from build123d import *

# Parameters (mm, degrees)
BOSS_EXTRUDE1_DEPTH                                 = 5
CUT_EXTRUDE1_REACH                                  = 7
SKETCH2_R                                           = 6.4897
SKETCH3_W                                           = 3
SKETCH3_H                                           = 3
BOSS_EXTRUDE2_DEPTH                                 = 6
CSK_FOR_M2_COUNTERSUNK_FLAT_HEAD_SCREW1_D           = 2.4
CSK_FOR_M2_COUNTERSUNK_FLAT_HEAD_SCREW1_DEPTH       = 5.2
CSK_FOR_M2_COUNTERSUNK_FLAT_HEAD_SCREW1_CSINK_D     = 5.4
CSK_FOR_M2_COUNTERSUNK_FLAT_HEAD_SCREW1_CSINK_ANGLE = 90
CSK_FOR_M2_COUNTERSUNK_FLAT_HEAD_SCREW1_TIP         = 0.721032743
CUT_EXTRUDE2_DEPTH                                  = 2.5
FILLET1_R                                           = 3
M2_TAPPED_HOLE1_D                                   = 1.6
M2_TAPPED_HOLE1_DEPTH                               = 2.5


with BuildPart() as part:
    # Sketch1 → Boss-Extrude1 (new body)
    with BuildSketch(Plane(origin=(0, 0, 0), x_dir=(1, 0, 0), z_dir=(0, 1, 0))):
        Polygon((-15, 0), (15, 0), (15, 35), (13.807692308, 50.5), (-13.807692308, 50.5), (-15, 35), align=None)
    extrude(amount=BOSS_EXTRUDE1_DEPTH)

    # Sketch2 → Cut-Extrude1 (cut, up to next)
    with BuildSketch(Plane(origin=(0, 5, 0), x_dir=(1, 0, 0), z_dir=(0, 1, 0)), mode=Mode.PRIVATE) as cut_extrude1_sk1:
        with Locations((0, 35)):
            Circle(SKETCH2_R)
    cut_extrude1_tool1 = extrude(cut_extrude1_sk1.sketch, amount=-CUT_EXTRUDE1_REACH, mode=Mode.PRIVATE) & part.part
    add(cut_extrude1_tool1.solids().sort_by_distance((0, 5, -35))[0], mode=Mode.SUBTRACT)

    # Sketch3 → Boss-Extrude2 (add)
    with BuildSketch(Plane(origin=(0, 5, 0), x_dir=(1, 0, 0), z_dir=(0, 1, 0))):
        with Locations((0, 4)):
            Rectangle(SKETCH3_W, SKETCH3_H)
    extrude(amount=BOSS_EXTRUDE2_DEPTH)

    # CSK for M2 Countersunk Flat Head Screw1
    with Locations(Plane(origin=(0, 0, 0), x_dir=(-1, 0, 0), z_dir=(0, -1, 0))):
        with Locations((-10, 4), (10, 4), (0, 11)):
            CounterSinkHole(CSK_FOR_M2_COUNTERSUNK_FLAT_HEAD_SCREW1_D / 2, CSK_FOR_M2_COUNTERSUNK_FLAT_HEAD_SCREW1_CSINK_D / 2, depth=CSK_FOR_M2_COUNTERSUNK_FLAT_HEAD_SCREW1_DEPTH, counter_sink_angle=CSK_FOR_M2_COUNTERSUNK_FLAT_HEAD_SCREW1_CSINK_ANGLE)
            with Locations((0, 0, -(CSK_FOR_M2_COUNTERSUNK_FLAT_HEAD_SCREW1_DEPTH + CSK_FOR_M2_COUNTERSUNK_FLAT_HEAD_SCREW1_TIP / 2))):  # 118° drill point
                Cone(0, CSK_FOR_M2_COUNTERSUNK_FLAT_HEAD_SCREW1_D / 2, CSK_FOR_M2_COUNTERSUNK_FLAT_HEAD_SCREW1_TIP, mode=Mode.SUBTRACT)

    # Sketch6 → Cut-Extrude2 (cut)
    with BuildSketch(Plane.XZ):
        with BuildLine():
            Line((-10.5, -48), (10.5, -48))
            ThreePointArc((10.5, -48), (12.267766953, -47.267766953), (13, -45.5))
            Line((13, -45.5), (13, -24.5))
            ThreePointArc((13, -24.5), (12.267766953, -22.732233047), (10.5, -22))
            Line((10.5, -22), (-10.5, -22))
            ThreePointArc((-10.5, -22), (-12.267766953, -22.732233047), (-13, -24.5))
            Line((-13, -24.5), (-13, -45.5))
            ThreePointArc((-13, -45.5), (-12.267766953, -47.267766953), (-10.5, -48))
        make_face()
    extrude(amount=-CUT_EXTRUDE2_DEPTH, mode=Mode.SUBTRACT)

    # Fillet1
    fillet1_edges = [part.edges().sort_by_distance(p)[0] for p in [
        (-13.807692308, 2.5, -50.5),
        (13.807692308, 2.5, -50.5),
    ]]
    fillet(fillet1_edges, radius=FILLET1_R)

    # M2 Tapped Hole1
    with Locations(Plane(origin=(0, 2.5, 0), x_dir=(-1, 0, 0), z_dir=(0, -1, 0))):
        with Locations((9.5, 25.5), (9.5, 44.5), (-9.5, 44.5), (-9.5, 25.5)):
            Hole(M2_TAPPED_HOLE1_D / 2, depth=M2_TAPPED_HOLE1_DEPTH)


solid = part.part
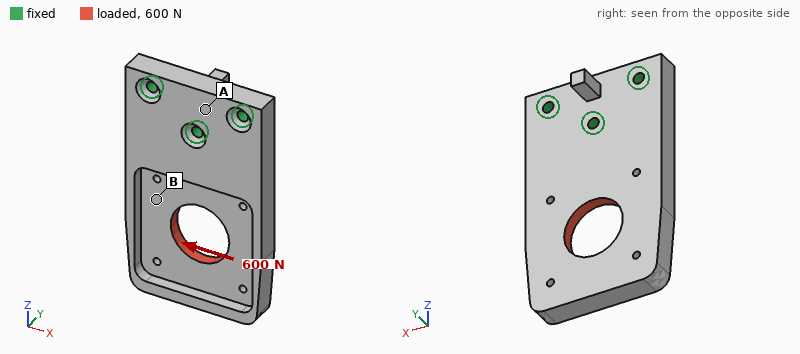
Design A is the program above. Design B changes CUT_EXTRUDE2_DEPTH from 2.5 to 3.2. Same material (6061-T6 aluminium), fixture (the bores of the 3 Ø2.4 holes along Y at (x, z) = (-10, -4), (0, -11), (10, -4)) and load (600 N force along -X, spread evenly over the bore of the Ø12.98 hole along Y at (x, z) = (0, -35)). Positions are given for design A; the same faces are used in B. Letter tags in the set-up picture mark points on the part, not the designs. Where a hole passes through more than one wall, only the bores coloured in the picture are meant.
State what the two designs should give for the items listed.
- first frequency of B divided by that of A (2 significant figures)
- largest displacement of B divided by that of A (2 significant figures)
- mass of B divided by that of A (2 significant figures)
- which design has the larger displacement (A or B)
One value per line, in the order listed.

1.0
1.3
0.93
B
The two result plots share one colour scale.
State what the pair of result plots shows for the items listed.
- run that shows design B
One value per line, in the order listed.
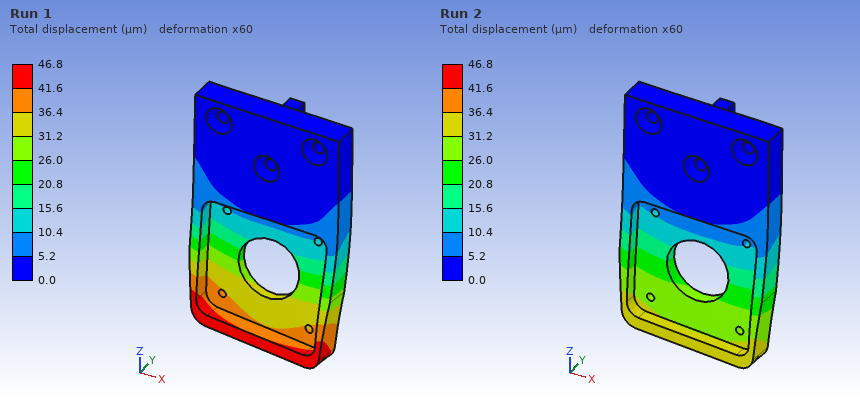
Run 1
